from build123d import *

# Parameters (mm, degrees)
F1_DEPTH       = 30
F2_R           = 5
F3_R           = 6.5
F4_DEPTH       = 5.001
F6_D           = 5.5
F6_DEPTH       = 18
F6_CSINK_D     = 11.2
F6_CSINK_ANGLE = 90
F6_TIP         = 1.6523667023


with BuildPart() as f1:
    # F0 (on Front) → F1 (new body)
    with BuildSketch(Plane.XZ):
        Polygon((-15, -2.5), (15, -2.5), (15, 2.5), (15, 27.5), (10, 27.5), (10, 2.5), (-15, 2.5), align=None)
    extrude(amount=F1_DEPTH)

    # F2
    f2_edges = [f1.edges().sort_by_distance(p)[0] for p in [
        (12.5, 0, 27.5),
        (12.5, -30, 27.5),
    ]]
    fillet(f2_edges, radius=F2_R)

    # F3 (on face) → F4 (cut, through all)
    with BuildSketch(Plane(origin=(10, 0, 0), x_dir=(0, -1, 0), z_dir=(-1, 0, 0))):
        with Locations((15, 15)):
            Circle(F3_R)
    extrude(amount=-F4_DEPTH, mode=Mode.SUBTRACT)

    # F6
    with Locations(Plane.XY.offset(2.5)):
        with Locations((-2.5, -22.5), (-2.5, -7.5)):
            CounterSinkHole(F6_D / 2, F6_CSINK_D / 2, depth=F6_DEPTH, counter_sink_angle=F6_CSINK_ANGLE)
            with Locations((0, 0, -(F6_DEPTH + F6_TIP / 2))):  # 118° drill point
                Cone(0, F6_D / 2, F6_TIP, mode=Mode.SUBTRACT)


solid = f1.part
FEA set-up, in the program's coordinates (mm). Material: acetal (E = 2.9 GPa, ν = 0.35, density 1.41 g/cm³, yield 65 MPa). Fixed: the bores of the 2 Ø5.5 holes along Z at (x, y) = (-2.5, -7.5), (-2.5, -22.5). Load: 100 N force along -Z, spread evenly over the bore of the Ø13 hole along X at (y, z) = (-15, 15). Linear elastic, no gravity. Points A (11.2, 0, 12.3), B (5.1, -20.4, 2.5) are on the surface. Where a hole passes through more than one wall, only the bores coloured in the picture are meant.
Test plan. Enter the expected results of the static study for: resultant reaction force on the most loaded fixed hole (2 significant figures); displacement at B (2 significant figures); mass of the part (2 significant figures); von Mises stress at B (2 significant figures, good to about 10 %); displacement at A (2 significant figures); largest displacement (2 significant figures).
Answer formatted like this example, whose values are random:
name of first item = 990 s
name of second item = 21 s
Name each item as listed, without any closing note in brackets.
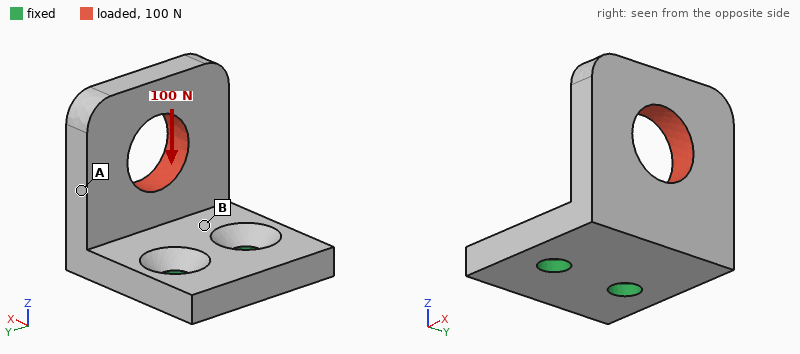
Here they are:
resultant reaction force on the most loaded fixed hole = 51 N
displacement at B = 0.099 mm
mass of the part = 10 g
von Mises stress at B = 5.1 MPa
displacement at A = 0.32 mm
largest displacement = 0.60 mm
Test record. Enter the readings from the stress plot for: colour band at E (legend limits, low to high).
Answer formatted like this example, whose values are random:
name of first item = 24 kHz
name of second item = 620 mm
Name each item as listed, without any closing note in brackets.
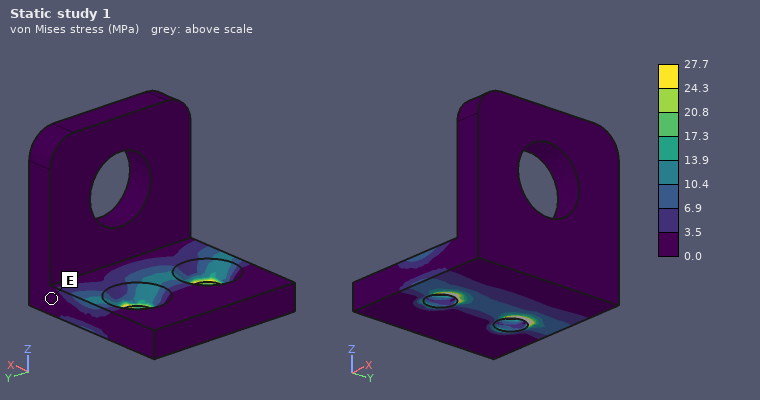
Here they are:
colour band at E = 0.0 to 3.5 MPa
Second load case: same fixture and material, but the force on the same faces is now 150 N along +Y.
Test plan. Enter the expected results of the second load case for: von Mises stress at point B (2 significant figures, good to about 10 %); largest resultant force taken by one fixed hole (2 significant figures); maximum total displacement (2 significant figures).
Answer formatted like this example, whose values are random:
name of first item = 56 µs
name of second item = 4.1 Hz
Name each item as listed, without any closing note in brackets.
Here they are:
von Mises stress at point B = 14 MPa
largest resultant force taken by one fixed hole = 200 N
maximum total displacement = 0.52 mm
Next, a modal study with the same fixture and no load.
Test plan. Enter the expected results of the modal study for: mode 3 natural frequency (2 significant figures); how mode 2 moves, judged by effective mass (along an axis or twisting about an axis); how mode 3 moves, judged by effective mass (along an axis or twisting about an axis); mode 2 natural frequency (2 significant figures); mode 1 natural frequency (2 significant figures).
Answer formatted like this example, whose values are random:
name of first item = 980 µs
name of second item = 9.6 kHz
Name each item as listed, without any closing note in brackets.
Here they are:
mode 3 natural frequency = 2400 Hz
how mode 2 moves, judged by effective mass = along Y
how mode 3 moves, judged by effective mass = along Z
mode 2 natural frequency = 1400 Hz
mode 1 natural frequency = 760 Hz
